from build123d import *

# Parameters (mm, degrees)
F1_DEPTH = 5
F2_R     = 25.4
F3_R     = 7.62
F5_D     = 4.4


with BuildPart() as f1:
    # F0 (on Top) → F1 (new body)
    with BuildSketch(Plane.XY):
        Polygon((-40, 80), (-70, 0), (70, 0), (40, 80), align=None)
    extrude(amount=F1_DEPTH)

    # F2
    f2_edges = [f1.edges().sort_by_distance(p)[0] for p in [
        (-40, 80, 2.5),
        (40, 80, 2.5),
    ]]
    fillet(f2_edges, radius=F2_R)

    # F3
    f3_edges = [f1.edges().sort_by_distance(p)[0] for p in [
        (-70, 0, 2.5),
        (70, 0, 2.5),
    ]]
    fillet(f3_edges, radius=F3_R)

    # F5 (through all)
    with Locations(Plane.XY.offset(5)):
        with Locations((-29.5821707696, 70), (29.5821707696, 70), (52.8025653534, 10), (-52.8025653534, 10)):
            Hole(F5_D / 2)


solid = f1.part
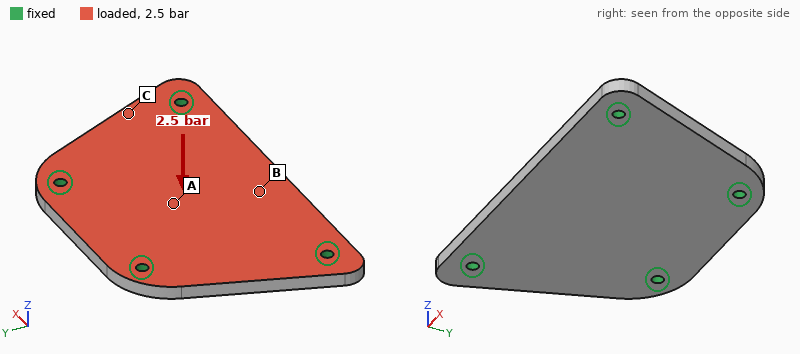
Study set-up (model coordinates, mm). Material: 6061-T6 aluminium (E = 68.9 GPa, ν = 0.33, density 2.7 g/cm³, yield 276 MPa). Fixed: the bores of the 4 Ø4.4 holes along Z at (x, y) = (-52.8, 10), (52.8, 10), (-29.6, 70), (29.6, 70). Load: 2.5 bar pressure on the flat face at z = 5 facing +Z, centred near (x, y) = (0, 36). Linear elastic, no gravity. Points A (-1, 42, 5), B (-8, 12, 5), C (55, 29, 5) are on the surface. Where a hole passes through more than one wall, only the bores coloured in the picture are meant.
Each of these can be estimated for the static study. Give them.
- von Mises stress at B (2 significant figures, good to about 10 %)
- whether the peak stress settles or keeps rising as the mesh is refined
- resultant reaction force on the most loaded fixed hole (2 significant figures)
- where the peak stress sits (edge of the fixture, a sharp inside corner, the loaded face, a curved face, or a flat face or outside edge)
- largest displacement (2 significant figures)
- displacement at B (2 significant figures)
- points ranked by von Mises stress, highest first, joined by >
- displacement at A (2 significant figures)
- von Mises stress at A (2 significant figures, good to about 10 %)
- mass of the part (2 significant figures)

23 MPa
keeps rising
560 N
edge of the fixture
0.13 mm
0.11 mm
B > A > C
0.071 mm
15 MPa
120 g
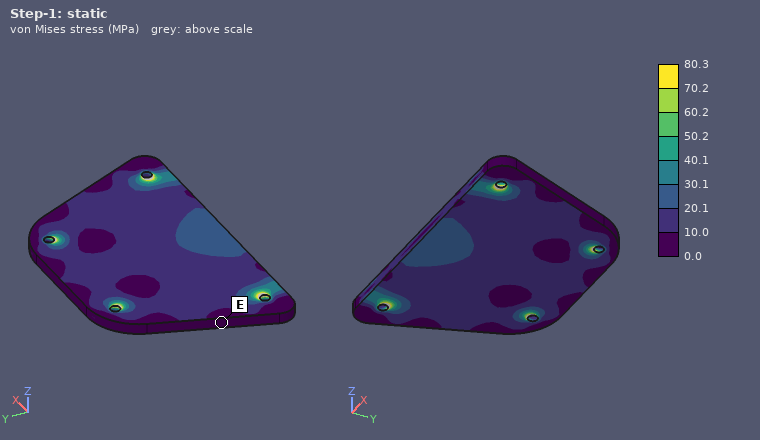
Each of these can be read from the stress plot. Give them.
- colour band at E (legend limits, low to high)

0.0 to 10.0 MPa
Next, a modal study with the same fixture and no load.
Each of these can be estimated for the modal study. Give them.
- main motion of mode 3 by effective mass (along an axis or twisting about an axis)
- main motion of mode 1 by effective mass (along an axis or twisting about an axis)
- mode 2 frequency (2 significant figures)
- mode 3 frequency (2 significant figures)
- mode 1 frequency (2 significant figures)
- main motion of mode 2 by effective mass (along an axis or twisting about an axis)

twisting about Y
along Z
5200 Hz
5600 Hz
2500 Hz
along Z
